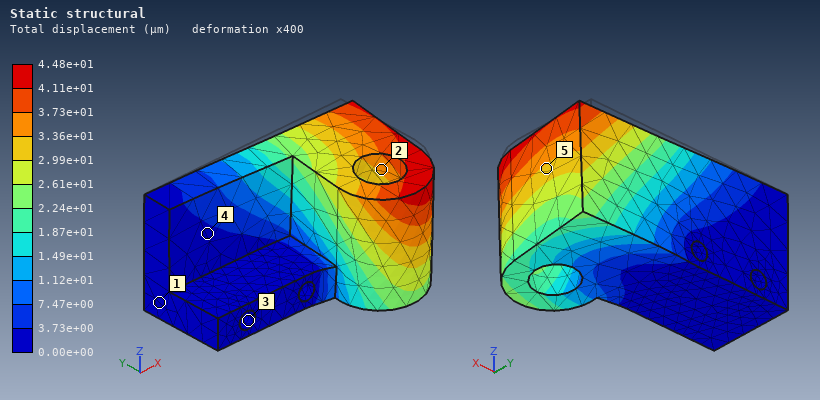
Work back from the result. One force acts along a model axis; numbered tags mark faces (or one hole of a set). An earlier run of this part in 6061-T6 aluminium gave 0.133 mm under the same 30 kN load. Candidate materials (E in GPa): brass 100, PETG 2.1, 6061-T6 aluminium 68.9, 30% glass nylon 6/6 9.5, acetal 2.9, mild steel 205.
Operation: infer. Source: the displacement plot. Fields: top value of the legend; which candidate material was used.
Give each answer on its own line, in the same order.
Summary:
4.48e+01 µm
mild steel
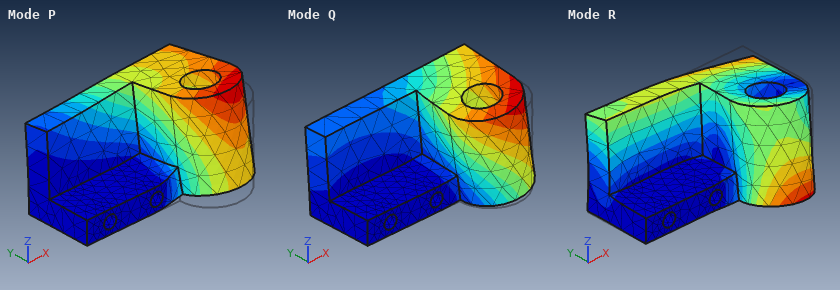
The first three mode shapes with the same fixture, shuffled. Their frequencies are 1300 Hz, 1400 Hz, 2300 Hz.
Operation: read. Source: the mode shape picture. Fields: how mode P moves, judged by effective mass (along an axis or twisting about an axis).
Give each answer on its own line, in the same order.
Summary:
along Y
